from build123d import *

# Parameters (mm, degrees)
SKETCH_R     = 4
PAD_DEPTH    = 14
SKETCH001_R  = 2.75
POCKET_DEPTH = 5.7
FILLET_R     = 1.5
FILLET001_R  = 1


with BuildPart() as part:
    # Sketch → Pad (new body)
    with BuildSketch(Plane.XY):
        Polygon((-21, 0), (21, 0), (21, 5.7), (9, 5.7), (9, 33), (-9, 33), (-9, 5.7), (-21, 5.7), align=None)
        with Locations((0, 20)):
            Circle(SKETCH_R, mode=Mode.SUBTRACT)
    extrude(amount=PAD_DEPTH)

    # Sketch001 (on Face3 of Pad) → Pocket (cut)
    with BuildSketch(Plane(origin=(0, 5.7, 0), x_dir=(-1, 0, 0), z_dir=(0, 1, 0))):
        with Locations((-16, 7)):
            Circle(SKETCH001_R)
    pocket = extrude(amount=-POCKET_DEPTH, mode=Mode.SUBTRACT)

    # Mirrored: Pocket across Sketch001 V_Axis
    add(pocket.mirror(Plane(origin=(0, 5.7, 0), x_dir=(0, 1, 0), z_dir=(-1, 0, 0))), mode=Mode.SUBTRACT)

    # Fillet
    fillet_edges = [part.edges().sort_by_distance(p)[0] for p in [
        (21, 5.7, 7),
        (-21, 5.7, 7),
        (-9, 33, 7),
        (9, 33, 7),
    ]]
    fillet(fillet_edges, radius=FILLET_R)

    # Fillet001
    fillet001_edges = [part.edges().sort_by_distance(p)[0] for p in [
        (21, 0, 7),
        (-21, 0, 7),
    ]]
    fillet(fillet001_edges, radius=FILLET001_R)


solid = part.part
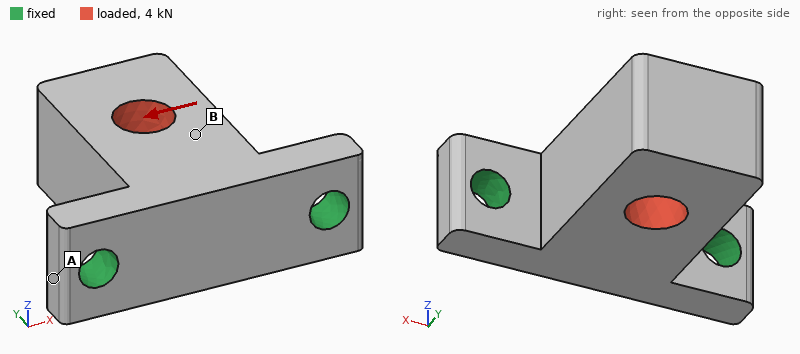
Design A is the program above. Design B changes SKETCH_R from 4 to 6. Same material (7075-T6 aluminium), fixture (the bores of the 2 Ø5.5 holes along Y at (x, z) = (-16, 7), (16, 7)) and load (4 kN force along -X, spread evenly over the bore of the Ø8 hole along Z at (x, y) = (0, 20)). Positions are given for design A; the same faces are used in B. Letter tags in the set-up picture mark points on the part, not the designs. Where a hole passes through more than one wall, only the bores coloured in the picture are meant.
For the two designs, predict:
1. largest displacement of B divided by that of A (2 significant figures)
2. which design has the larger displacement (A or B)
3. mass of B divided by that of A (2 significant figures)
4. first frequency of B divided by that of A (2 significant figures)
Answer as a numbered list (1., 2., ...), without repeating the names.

1. 1.3
2. B
3. 0.90
4. 1.0
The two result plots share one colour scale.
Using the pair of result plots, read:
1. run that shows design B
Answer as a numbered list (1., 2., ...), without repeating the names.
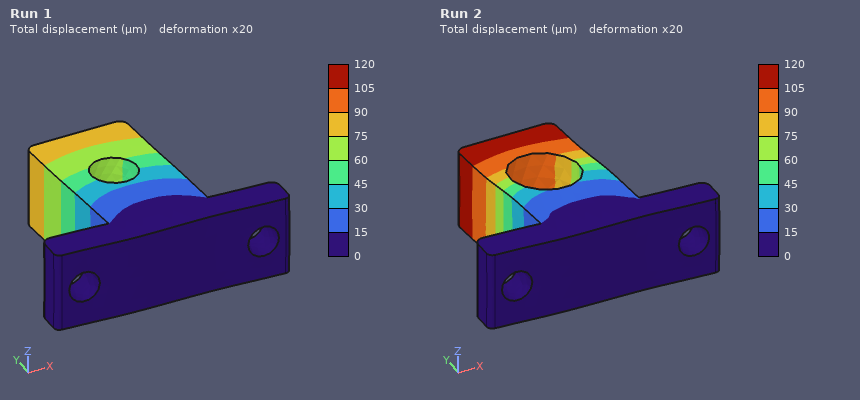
1. Run 2
